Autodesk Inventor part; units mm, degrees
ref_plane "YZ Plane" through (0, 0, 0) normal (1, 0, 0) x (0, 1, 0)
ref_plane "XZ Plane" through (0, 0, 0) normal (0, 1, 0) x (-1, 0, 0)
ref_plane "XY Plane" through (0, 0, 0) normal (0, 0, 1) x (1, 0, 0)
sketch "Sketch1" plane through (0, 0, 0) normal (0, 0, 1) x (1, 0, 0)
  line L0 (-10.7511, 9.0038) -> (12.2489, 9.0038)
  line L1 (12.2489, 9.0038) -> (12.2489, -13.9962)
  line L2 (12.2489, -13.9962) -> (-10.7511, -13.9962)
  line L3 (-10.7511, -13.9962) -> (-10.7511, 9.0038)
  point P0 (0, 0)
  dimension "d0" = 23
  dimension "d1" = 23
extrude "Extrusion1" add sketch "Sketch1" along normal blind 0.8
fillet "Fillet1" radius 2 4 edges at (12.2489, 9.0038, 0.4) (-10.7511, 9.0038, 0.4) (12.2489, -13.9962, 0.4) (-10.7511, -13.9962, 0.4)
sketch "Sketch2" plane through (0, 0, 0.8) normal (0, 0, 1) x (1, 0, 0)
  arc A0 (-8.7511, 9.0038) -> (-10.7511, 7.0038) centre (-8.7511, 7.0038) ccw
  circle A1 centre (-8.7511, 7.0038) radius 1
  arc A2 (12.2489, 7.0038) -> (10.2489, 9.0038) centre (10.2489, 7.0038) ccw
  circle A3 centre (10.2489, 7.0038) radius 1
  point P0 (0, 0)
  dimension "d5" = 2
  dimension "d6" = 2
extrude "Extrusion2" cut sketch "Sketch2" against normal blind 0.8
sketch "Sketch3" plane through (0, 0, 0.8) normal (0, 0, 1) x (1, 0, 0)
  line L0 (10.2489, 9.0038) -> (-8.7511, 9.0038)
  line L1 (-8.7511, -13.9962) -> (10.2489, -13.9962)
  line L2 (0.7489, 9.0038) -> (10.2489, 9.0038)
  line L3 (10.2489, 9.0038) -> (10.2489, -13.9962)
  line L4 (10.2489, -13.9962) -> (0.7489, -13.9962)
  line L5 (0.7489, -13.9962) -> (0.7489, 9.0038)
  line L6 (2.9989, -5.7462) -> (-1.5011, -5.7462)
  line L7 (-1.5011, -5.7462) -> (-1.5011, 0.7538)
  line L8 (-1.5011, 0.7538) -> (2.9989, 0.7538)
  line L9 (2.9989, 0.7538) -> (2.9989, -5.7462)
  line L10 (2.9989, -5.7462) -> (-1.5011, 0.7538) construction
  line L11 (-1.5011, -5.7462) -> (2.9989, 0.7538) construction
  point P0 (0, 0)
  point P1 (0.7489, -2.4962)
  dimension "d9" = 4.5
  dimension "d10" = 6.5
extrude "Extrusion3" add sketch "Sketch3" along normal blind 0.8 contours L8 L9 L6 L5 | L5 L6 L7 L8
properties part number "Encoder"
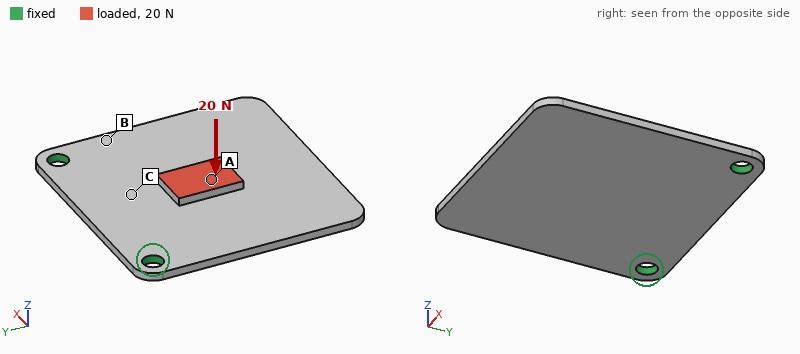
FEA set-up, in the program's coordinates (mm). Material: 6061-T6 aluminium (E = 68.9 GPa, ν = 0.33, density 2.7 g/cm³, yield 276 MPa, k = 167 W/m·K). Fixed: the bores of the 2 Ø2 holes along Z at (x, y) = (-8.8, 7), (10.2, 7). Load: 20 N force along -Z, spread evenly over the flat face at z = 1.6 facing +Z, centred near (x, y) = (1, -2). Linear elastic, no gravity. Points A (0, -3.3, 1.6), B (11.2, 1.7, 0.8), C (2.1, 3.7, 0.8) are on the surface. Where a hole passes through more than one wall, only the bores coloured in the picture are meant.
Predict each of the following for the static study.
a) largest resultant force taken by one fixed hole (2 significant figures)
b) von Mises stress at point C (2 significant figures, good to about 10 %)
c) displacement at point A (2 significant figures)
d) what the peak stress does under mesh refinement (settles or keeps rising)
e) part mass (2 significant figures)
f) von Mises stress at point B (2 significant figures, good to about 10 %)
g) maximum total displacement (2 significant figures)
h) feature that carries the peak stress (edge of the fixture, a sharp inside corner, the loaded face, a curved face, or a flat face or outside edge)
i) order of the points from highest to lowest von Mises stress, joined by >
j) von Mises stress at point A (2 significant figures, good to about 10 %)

10 N
31 MPa
0.14 mm
keeps rising
1.2 g
48 MPa
0.32 mm
edge of the fixture
B > C > A
14 MPa
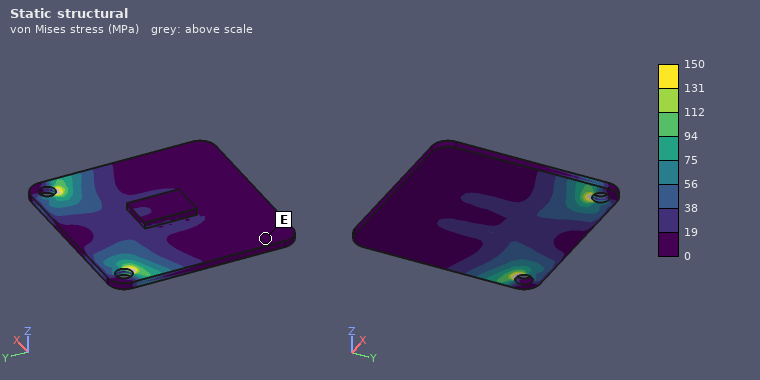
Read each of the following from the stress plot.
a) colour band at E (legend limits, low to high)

0 to 19 MPa
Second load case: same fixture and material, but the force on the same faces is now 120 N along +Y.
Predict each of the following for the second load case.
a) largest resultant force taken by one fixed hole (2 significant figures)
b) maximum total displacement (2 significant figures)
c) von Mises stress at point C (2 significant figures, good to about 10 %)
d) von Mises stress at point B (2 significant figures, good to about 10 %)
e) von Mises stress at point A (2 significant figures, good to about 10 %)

65 N
0.34 mm
48 MPa
61 MPa
21 MPa
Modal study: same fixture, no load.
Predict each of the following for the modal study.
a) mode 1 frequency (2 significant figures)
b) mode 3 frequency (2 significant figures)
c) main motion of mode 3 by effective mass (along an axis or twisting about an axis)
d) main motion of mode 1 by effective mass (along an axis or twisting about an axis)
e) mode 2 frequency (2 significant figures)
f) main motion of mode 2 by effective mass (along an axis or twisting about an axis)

1400 Hz
8900 Hz
along Z
along Z
4000 Hz
twisting about Y
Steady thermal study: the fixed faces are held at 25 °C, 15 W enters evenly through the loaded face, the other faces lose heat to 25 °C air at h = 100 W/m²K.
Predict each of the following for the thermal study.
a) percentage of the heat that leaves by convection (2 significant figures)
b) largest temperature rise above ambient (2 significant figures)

25 %
60 K
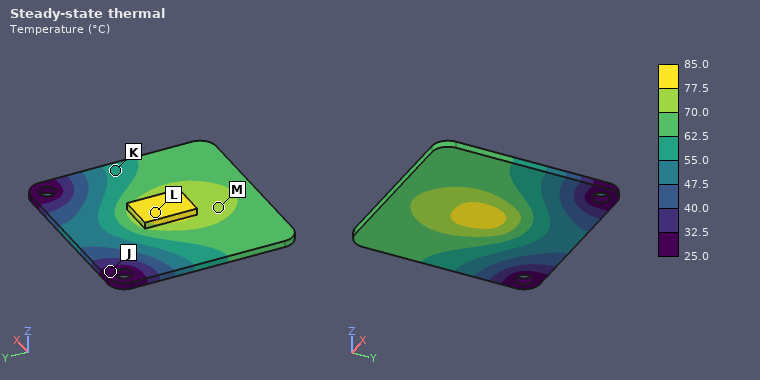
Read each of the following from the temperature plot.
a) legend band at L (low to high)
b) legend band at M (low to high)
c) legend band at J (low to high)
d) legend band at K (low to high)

77.5 to 85.0 °C
70.0 to 77.5 °C
25.0 to 32.5 °C
55.0 to 62.5 °C
